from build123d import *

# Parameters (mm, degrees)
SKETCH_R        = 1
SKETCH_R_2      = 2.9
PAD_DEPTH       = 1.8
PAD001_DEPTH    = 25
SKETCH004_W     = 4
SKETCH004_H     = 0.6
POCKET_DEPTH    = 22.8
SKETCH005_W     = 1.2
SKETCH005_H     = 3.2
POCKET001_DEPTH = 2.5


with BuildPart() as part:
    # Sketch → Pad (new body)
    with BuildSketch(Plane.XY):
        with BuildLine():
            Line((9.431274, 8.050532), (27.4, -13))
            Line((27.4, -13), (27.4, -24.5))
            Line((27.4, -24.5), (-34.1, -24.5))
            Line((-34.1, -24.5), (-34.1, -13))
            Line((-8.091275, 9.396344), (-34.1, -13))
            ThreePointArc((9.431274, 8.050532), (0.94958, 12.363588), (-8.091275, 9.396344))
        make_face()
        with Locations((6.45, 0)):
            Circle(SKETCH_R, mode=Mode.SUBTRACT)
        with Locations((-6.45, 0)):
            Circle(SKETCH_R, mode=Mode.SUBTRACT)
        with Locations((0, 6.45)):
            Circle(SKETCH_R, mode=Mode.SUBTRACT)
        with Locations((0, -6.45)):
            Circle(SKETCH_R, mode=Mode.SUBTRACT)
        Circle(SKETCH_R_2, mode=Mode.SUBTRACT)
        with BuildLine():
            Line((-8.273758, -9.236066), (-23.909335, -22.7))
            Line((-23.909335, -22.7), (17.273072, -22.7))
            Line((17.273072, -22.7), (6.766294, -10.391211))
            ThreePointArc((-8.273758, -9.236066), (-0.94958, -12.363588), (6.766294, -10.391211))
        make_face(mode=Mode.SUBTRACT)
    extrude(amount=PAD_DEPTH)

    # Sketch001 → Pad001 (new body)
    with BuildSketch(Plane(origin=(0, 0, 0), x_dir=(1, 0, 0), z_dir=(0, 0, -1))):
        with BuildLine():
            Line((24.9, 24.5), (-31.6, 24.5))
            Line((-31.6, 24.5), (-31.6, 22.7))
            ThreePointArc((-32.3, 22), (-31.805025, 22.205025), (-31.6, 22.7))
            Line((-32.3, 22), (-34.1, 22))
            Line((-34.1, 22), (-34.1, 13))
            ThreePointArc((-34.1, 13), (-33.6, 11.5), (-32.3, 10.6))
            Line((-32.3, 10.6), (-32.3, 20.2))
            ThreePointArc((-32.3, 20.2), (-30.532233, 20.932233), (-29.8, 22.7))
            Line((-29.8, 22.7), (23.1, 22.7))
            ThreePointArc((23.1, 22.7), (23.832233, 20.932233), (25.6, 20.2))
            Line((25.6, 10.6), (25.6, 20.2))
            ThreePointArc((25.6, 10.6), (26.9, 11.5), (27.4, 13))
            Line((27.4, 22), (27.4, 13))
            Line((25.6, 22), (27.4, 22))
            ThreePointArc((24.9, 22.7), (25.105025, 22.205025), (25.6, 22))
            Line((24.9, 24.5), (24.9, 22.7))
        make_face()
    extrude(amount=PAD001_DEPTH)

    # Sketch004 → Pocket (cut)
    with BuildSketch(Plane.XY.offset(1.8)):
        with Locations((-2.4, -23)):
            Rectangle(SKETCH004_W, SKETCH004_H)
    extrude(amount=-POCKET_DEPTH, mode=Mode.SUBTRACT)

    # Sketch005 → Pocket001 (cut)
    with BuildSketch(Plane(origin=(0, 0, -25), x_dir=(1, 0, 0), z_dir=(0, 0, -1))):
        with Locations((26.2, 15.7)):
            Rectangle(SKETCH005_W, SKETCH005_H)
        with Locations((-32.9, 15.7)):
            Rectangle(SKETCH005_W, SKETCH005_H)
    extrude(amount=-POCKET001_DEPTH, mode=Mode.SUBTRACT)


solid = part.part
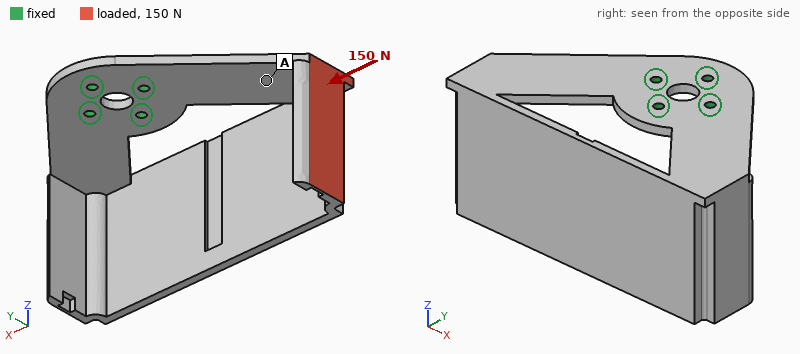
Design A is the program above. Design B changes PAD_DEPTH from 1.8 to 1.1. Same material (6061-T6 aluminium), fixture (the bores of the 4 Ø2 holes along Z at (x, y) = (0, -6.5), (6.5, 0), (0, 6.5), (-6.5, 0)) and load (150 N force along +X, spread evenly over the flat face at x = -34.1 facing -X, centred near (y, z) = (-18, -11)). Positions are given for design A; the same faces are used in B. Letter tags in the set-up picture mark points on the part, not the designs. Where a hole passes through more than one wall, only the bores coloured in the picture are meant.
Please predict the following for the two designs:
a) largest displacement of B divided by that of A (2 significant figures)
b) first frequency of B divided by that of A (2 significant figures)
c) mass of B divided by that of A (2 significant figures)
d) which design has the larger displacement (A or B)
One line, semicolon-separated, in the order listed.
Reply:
2.9; 0.51; 0.85; B
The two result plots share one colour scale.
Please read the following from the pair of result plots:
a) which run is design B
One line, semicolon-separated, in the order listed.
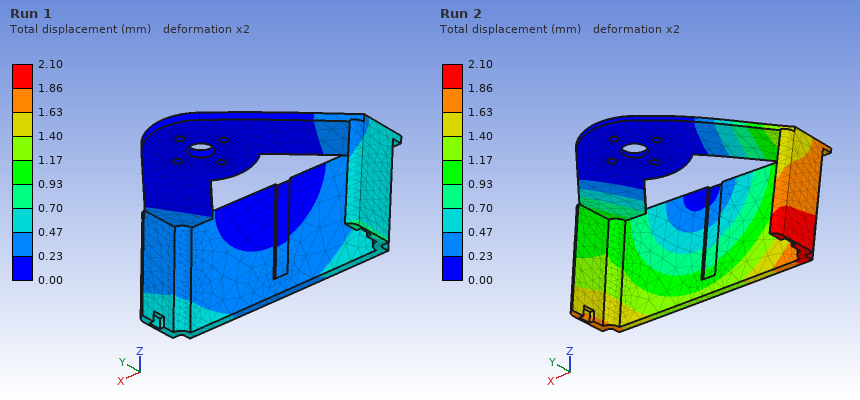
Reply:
Run 2
